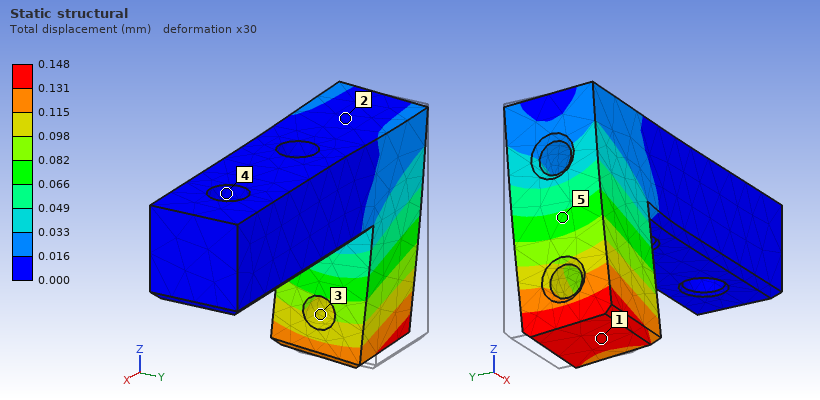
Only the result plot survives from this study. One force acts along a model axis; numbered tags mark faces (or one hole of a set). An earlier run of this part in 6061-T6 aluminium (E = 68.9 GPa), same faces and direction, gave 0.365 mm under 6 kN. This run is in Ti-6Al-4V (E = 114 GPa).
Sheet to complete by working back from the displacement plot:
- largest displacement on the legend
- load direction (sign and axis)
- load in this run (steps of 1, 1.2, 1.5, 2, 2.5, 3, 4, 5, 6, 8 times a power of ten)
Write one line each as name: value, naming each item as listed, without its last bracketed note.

largest displacement on the legend: 0.148 mm
load direction: -Y
load in this run: 4 kN
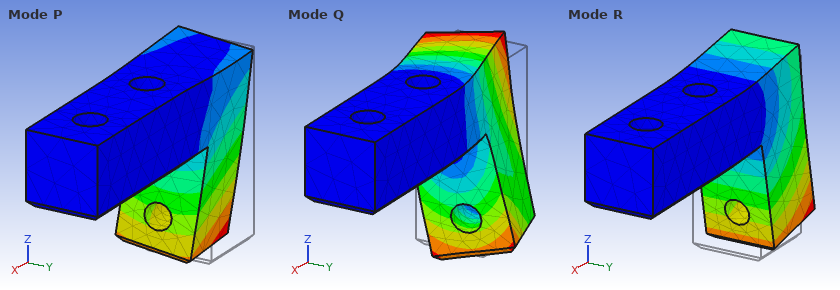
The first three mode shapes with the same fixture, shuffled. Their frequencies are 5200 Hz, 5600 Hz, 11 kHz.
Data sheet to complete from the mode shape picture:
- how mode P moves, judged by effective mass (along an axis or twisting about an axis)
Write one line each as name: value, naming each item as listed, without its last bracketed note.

how mode P moves, judged by effective mass: along Y
